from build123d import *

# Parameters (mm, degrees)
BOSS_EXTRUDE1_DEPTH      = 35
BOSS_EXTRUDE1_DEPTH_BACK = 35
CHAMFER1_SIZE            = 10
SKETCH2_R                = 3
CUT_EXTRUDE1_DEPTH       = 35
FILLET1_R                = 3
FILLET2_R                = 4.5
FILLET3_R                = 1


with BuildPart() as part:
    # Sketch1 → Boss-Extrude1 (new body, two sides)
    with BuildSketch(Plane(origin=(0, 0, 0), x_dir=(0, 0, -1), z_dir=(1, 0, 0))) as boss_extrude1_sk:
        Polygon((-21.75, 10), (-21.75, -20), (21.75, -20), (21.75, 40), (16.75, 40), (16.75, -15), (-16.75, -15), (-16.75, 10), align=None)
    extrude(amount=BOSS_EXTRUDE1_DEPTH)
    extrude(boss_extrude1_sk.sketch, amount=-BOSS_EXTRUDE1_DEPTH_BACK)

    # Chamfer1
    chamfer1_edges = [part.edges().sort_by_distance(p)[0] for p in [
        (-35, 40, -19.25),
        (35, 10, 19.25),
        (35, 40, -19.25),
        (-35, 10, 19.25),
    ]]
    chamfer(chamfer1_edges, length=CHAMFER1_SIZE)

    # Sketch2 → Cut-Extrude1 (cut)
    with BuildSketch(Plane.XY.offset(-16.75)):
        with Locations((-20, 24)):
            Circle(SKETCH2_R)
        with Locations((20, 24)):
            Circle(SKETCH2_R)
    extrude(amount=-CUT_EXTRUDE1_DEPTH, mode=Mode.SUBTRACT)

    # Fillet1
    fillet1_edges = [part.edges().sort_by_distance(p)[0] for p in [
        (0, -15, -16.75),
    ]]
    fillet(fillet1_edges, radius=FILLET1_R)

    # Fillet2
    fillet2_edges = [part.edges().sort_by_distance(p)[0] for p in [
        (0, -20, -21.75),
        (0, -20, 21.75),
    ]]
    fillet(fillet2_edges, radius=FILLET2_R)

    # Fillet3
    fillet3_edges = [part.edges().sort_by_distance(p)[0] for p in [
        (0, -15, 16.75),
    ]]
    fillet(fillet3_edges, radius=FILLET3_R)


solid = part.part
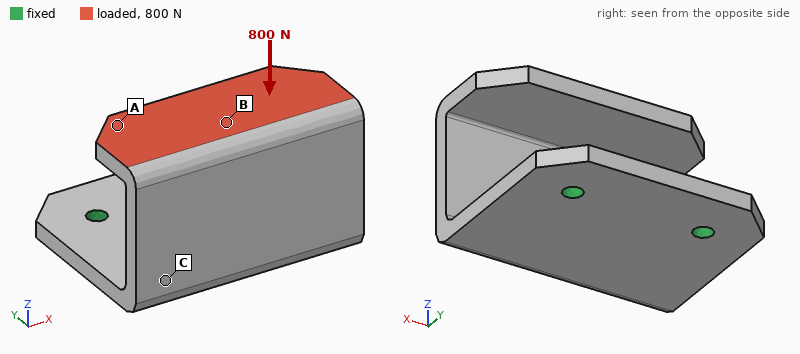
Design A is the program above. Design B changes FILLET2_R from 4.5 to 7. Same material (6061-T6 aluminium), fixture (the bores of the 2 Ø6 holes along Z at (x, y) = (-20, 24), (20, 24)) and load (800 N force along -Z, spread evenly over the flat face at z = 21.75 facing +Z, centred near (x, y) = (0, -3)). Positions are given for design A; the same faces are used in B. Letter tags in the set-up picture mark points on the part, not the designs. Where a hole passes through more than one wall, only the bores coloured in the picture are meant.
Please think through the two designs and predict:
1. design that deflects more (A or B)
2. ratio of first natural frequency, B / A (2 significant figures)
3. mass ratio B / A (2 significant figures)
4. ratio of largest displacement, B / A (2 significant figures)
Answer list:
B
1.0
0.98
1.1
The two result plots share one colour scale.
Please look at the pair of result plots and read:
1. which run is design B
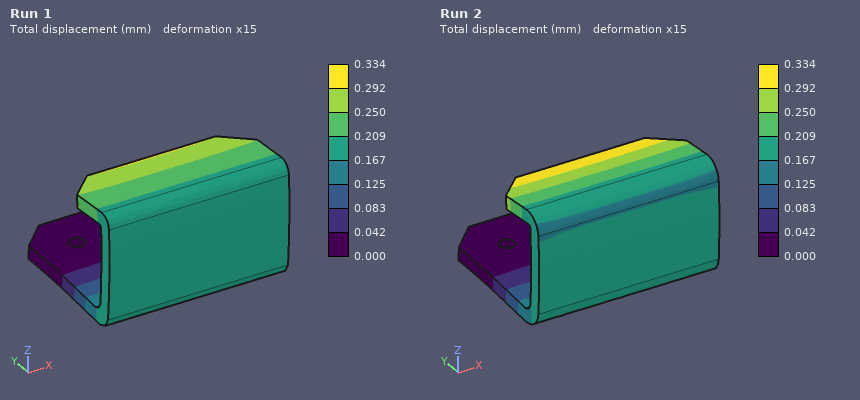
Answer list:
Run 2
